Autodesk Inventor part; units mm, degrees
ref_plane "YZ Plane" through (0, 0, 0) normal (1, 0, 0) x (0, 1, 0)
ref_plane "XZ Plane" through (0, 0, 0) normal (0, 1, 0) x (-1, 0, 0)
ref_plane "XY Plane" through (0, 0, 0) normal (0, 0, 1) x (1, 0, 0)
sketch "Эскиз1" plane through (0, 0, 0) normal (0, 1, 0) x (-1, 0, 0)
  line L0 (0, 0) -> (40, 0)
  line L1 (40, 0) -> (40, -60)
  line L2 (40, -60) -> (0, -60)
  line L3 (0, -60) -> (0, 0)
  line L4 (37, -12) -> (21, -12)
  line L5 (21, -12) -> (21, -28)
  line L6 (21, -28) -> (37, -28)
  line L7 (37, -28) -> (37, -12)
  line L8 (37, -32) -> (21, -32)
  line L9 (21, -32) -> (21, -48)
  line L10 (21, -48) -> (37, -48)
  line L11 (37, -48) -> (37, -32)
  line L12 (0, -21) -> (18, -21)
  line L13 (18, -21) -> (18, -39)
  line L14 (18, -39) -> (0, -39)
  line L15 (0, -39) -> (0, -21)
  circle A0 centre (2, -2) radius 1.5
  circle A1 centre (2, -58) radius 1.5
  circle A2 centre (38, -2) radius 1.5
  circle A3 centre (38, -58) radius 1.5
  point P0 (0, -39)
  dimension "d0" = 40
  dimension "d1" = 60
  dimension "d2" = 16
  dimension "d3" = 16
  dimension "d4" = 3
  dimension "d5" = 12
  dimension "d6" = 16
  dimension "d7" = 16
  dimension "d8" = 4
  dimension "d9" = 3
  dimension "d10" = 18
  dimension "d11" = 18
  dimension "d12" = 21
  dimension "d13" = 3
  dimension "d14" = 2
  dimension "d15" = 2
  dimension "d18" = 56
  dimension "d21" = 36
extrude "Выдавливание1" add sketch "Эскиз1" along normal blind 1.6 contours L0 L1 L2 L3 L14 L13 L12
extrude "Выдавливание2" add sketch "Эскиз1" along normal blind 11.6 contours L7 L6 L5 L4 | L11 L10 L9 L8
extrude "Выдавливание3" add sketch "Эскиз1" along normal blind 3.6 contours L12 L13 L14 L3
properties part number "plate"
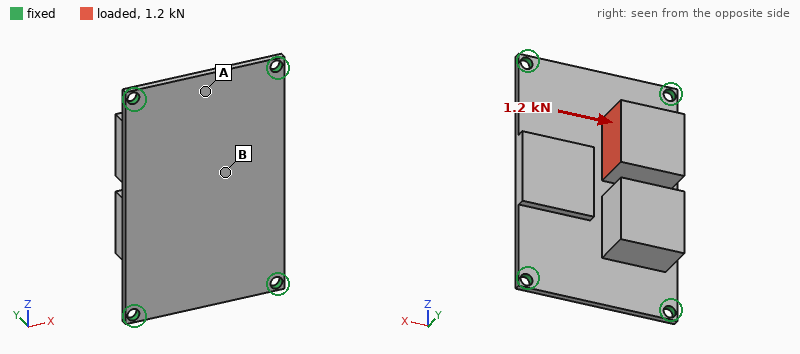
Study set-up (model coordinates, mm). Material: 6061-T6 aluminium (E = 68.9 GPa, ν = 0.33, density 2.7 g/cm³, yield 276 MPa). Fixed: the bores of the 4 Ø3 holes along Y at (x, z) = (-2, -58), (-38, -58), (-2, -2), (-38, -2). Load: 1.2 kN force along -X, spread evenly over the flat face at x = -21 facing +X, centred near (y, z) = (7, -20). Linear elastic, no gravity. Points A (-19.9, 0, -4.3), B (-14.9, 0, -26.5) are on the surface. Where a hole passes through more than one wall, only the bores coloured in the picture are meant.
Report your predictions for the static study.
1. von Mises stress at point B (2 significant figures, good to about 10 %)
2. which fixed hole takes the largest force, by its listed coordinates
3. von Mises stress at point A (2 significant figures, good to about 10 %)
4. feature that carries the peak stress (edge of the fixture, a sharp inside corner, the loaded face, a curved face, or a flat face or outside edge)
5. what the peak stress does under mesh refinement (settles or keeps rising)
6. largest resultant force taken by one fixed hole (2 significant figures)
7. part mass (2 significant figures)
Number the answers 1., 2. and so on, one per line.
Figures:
1. 25 MPa
2. (-38, -2)
3. 71 MPa
4. edge of the fixture
5. keeps rising
6. 510 N
7. 26 g
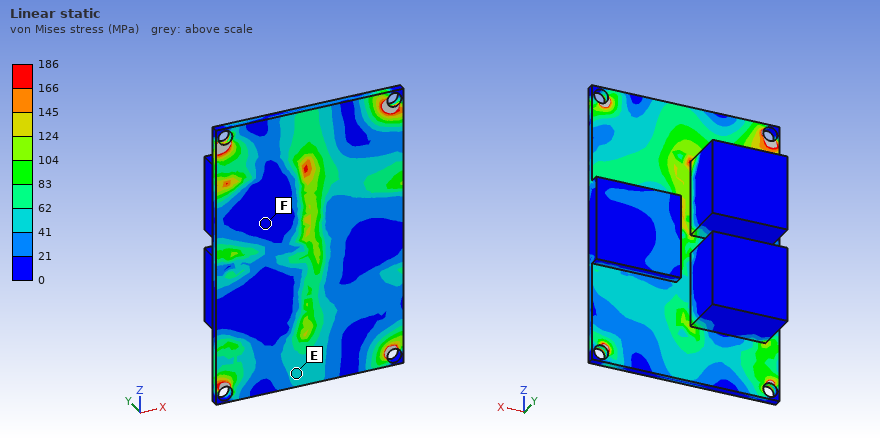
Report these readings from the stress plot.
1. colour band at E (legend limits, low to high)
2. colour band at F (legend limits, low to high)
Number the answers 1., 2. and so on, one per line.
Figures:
1. 41 to 62 MPa
2. 0 to 21 MPa
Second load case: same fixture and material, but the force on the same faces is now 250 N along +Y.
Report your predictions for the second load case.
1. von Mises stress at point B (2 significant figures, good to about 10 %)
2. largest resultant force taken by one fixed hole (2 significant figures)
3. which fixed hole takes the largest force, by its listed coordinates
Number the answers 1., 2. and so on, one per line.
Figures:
1. 21 MPa
2. 110 N
3. (-38, -2)
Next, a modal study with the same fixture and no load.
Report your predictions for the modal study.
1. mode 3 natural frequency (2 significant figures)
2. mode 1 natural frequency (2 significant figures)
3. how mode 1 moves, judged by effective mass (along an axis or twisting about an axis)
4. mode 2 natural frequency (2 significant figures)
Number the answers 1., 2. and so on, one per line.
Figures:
1. 4800 Hz
2. 1700 Hz
3. along Y
4. 3000 Hz
